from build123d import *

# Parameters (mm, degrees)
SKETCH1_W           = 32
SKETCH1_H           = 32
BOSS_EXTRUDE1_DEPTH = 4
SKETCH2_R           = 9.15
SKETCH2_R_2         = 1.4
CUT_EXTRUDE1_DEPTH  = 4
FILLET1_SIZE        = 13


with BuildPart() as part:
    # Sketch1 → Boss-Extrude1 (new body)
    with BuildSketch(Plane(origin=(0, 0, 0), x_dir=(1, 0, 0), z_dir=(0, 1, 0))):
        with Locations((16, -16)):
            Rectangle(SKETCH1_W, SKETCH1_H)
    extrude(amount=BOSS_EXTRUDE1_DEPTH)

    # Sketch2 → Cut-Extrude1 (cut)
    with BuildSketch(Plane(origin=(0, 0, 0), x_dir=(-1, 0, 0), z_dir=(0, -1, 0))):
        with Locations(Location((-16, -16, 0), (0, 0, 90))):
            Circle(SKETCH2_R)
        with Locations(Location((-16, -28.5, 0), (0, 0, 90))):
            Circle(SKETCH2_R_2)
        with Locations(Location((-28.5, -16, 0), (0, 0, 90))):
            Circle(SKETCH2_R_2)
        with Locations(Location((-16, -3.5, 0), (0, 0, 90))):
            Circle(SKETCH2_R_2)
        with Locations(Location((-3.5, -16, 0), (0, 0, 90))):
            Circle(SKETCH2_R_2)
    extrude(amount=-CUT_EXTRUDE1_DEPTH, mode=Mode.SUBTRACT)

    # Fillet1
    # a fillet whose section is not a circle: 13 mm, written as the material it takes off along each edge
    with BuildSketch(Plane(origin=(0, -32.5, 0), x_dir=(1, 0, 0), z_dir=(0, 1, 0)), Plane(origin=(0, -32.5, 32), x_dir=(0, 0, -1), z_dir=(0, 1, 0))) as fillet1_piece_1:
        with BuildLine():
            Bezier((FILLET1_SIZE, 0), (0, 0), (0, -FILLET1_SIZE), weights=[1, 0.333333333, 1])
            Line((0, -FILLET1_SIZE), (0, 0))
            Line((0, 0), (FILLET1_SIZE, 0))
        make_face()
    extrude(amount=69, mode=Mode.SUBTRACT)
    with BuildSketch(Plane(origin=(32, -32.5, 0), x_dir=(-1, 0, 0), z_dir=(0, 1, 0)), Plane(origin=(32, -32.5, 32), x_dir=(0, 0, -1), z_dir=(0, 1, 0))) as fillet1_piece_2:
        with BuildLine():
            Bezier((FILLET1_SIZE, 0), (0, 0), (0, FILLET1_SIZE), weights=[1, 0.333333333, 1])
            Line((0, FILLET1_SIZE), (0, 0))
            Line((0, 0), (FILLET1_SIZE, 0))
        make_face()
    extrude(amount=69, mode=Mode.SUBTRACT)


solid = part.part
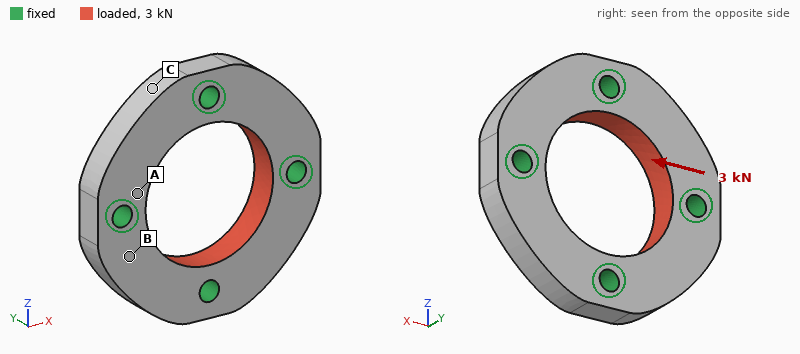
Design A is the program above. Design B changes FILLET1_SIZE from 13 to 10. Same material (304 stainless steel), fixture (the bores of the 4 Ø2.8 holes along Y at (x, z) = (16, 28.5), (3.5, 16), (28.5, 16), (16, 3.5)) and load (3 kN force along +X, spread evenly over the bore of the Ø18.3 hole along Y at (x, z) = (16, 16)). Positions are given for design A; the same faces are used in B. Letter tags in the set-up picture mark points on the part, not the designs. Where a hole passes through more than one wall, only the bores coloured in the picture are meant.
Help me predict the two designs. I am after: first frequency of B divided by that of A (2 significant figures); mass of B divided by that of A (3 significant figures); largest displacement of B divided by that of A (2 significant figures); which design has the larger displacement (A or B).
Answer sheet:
0.82
1.17
0.87
A
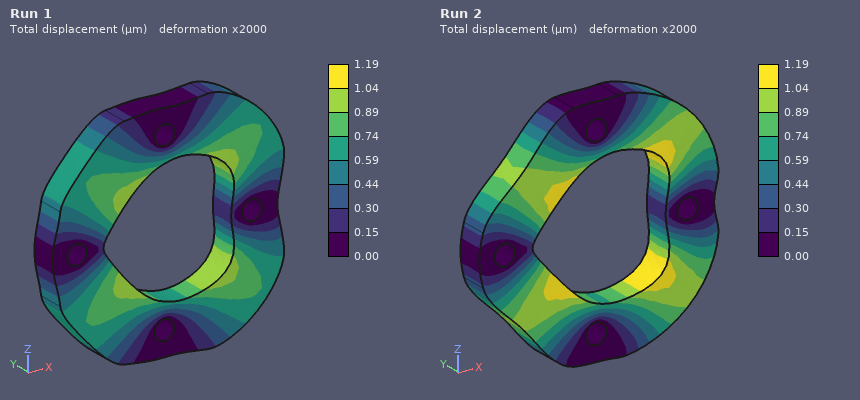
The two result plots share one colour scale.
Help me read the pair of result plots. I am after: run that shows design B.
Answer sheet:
Run 1
